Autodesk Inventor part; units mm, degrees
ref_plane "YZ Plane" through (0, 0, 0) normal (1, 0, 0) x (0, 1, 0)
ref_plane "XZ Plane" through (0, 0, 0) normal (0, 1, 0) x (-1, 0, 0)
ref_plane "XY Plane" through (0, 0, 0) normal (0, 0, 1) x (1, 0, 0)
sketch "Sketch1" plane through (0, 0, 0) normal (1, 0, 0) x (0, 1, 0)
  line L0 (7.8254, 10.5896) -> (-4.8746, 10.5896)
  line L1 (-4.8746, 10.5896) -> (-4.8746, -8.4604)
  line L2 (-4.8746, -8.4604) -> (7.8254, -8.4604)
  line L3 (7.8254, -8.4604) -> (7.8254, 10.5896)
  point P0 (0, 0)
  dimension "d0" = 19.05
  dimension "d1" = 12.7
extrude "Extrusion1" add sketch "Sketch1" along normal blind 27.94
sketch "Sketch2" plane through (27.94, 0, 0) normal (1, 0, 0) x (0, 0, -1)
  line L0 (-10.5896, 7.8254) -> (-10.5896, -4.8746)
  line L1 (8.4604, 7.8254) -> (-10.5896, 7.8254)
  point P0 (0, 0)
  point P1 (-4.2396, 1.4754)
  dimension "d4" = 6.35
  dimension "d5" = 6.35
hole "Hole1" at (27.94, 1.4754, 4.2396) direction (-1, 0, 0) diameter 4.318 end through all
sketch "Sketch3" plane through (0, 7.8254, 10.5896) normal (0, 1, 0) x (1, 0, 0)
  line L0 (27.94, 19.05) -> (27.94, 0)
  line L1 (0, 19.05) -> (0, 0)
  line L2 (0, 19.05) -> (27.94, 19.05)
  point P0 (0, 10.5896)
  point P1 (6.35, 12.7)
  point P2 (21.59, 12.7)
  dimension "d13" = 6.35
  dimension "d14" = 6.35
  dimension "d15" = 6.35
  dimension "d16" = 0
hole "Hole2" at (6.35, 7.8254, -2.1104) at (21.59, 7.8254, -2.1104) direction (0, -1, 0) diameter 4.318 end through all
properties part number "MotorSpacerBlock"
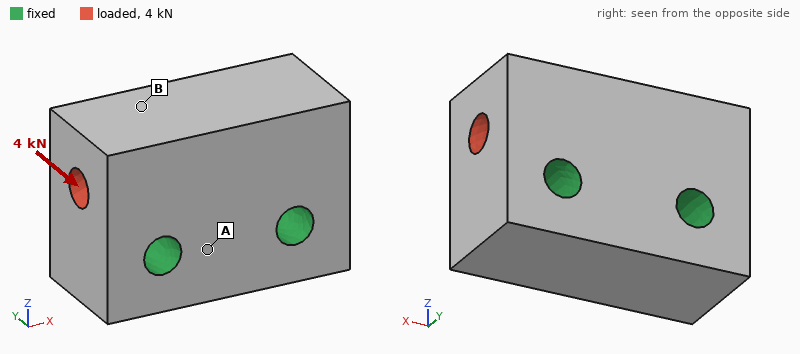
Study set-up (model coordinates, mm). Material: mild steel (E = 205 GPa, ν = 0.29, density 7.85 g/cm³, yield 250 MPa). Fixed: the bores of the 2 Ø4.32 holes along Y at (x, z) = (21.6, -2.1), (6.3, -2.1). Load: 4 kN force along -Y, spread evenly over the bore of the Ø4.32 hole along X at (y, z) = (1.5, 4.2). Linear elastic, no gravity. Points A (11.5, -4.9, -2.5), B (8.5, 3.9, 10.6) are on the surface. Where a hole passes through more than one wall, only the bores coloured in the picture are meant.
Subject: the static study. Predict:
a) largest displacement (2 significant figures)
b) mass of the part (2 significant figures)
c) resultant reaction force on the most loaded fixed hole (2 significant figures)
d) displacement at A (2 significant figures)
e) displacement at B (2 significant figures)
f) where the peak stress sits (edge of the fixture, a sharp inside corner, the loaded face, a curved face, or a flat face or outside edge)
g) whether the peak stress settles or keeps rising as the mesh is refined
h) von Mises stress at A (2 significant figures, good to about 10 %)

2.7 µm
47 g
2.0 kN
0.52 µm
2.5 µm
edge of the fixture
keeps rising
15 MPa
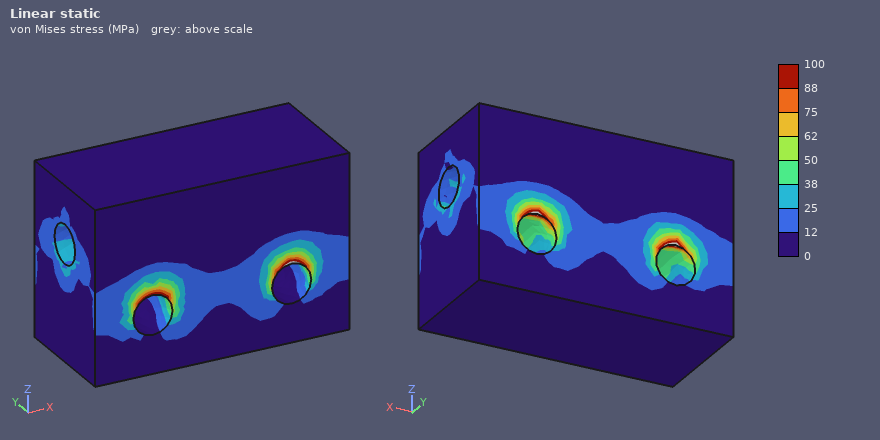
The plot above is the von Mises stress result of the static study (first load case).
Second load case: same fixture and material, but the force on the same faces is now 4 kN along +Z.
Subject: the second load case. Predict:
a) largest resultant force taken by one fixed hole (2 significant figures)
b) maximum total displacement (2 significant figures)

2.0 kN
0.80 µm
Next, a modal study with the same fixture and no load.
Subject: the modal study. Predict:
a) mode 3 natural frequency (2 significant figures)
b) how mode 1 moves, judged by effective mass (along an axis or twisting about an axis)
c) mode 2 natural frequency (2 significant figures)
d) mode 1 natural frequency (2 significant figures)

49 kHz
along Y
48 kHz
38 kHz
